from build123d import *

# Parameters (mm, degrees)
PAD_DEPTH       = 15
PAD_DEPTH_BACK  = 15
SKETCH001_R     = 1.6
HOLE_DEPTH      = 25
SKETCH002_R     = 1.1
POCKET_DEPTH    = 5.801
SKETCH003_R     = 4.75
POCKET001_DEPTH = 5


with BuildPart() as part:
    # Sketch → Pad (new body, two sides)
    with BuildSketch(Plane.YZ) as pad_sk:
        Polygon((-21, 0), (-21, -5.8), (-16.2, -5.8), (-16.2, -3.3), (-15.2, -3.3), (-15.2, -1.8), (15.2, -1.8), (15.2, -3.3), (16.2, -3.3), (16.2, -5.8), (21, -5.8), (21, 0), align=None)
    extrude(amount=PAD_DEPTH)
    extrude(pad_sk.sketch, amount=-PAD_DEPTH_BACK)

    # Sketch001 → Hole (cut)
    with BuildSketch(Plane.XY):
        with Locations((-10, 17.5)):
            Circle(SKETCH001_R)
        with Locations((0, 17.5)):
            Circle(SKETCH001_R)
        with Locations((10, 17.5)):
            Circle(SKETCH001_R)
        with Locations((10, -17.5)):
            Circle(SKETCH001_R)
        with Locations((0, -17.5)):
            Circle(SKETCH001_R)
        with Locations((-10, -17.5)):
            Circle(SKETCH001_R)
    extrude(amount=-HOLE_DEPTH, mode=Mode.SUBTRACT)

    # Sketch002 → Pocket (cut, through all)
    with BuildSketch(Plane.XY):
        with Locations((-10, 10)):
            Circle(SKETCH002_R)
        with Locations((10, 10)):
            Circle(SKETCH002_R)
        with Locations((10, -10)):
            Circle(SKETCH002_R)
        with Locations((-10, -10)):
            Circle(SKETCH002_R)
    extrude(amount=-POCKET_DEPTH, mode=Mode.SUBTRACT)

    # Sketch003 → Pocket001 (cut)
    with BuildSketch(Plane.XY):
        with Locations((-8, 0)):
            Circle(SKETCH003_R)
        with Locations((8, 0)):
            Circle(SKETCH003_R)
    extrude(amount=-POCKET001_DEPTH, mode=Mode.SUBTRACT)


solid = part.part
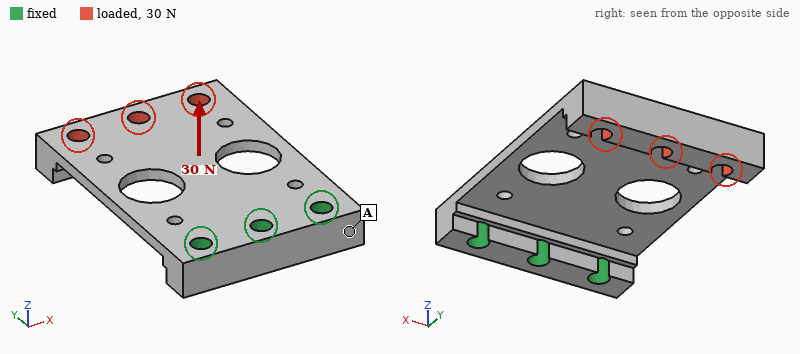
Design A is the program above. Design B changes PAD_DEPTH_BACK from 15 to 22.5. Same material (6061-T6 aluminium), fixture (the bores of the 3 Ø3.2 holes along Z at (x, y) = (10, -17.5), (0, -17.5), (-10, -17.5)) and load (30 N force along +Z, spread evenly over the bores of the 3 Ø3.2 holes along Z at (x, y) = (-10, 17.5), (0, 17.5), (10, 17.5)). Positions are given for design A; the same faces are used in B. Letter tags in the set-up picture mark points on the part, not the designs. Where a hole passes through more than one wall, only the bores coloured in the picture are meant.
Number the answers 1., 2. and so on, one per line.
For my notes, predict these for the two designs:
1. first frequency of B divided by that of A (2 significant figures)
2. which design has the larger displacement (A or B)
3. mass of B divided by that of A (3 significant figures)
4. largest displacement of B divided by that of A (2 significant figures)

1. 1.0
2. A
3. 1.30
4. 0.77
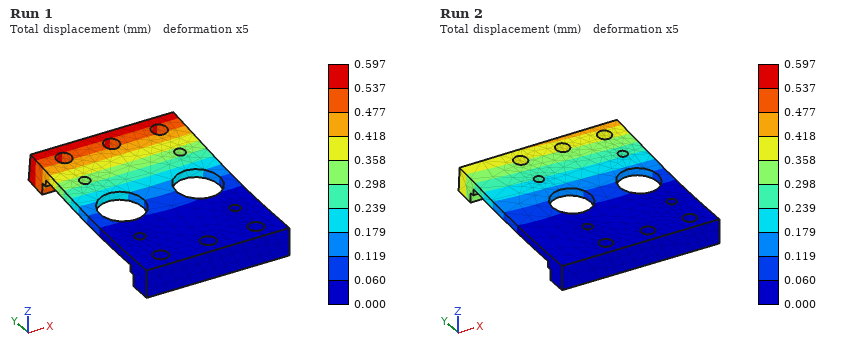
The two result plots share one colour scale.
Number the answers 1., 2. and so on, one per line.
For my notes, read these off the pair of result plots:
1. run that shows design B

1. Run 2
